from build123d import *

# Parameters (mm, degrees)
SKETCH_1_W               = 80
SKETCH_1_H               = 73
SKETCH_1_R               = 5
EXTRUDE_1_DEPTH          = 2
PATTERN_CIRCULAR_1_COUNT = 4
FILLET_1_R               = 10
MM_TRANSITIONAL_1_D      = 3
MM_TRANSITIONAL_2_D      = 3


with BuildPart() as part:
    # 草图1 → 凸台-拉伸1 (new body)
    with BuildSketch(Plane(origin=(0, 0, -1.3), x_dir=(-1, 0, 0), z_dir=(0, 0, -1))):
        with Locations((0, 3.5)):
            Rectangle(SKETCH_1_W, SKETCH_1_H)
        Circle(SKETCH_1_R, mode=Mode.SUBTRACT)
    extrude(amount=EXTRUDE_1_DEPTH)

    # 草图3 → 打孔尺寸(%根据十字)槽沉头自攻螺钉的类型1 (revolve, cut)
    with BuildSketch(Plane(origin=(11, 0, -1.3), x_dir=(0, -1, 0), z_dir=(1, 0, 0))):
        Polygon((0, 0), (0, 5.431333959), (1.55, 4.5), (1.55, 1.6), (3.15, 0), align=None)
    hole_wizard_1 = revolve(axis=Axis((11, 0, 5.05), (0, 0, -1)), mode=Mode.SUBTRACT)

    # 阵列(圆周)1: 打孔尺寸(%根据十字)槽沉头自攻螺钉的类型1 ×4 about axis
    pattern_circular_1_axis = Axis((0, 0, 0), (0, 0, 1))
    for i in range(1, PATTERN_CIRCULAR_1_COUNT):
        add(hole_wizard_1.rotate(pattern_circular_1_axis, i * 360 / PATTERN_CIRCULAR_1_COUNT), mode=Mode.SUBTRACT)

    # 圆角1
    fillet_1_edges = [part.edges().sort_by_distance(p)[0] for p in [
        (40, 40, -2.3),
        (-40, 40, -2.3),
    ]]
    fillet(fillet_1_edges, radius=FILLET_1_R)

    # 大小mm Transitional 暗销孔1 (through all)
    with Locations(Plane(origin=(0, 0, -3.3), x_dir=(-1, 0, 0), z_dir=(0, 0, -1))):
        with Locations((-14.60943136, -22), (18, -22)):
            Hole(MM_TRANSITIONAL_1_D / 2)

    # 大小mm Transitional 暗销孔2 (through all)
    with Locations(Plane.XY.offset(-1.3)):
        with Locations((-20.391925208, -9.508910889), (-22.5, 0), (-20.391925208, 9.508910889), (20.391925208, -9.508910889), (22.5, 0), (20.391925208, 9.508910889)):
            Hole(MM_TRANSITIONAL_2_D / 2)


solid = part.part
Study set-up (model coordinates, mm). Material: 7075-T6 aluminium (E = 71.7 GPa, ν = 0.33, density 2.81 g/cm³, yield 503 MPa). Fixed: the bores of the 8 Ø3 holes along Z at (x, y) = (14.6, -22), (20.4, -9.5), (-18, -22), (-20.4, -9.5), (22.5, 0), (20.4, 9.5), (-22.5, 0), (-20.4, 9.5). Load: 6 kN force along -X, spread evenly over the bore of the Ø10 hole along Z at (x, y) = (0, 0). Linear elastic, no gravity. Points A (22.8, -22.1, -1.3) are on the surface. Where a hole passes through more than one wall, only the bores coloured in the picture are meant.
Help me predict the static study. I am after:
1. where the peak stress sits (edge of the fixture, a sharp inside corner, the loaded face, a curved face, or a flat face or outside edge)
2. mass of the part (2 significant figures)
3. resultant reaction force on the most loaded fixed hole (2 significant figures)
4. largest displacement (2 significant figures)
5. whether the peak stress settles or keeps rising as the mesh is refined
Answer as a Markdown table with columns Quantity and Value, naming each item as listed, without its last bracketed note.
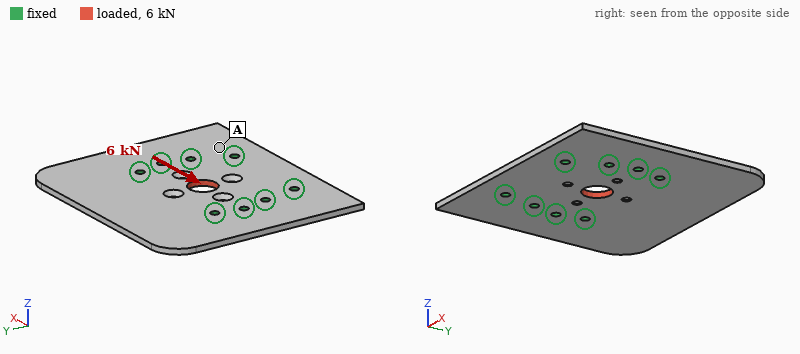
| Quantity | Value |
|---|---|
| where the peak stress sits | a sharp inside corner |
| mass of the part | 31 g |
| resultant reaction force on the most loaded fixed hole | 1.2 kN |
| largest displacement | 22 µm |
| whether the peak stress settles or keeps rising as the mesh is refined | keeps rising |
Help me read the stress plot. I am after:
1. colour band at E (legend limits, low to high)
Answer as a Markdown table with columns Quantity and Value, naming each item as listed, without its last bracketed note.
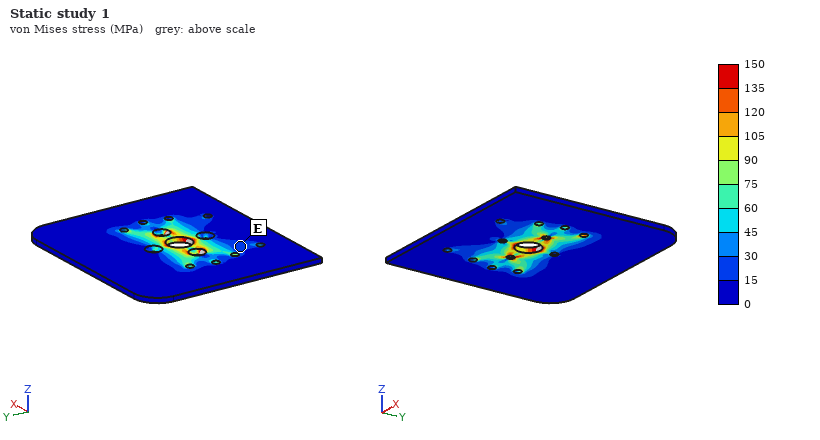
| Quantity | Value |
|---|---|
| colour band at E | 15 to 30 MPa |
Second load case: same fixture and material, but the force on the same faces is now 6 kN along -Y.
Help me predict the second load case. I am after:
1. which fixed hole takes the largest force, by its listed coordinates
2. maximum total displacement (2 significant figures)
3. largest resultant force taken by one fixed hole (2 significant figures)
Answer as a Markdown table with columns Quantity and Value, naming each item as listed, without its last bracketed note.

| Quantity | Value |
|---|---|
| which fixed hole takes the largest force, by its listed coordinates | (14.6, -22) |
| maximum total displacement | 31 µm |
| largest resultant force taken by one fixed hole | 1.3 kN |
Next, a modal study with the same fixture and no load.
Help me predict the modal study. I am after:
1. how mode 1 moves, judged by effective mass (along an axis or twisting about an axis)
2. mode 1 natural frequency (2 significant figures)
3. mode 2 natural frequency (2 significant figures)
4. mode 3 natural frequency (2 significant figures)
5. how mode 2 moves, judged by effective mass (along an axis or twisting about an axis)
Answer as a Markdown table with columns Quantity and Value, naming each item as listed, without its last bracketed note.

| Quantity | Value |
|---|---|
| how mode 1 moves, judged by effective mass | along Z |
| mode 1 natural frequency | 1600 Hz |
| mode 2 natural frequency | 2100 Hz |
| mode 3 natural frequency | 3000 Hz |
| how mode 2 moves, judged by effective mass | twisting about Y |
